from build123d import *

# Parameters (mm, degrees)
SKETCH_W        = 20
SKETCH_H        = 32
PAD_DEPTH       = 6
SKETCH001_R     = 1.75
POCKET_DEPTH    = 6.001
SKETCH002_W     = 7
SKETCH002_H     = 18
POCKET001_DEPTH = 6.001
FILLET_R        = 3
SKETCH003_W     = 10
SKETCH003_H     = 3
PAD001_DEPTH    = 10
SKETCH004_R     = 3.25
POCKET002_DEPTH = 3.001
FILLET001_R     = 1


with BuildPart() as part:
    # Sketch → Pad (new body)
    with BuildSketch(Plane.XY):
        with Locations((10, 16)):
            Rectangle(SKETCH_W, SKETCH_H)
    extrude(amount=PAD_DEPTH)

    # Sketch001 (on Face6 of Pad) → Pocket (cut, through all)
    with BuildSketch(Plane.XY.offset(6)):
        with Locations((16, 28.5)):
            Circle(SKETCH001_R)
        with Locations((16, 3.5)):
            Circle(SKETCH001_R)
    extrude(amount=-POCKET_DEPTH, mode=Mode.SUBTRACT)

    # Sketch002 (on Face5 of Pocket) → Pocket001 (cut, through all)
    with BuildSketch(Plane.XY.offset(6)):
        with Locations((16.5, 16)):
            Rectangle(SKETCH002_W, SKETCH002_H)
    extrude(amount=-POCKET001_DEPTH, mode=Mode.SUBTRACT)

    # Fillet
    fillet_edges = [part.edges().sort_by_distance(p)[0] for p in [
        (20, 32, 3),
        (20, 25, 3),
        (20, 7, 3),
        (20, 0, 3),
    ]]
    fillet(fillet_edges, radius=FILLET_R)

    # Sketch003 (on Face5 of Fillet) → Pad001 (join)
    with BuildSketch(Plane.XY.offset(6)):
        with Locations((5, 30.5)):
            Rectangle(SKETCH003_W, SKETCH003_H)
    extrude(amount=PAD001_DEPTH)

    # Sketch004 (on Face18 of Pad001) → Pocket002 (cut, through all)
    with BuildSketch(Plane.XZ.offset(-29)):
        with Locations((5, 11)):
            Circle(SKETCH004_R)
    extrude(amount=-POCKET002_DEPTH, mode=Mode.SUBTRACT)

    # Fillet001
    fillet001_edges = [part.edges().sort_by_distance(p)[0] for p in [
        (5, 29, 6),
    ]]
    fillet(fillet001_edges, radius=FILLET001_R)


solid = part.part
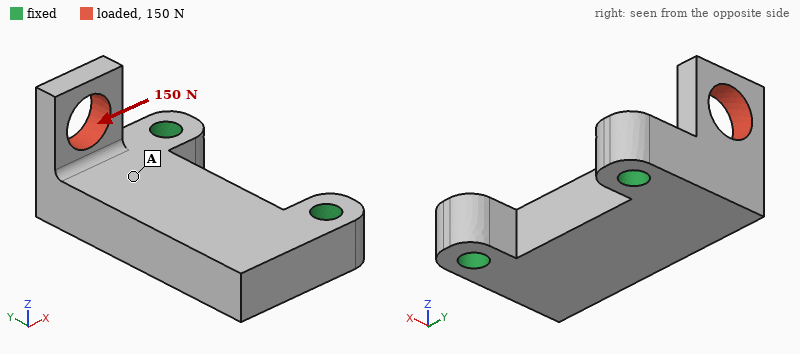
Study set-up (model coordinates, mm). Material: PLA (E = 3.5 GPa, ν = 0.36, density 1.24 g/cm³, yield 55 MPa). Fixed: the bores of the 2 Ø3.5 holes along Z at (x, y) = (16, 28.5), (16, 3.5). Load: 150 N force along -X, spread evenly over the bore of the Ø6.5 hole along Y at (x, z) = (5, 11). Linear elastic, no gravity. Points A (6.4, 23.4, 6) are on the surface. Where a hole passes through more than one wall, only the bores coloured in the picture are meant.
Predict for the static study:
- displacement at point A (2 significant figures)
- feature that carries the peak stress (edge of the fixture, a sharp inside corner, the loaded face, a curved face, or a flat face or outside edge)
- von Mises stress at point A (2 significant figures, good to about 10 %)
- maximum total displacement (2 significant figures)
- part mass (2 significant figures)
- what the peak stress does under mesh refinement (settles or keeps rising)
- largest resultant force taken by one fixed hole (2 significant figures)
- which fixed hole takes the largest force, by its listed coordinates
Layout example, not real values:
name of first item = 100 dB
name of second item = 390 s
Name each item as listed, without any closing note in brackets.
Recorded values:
displacement at point A = 0.075 mm
feature that carries the peak stress = a sharp inside corner
von Mises stress at point A = 6.3 MPa
maximum total displacement = 0.47 mm
part mass = 3.9 g
what the peak stress does under mesh refinement = keeps rising
largest resultant force taken by one fixed hole = 160 N
which fixed hole takes the largest force, by its listed coordinates = (16, 28.5)
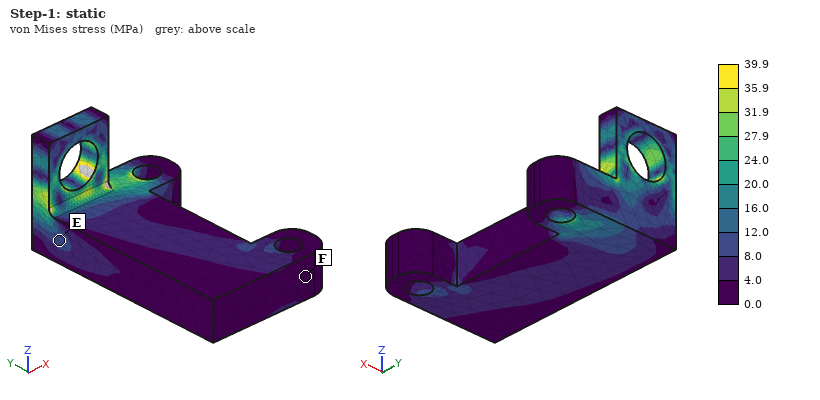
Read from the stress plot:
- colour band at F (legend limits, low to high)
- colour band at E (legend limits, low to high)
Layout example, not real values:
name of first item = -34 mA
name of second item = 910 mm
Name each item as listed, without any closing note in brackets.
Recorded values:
colour band at F = 0.0 to 4.0 MPa
colour band at E = 8.0 to 12.0 MPa
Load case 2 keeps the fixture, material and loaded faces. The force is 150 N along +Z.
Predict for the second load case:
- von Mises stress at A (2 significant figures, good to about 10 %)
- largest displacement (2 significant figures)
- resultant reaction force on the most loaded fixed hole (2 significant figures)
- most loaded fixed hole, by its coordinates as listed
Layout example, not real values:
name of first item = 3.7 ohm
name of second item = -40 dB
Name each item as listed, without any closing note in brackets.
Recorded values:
von Mises stress at A = 5.2 MPa
largest displacement = 0.28 mm
resultant reaction force on the most loaded fixed hole = 150 N
most loaded fixed hole, by its coordinates as listed = (16, 28.5)
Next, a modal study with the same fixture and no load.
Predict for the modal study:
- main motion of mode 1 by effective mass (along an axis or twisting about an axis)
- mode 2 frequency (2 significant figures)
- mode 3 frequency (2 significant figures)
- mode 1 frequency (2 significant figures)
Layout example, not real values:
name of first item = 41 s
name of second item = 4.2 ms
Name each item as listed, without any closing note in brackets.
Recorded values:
main motion of mode 1 by effective mass = along Z
mode 2 frequency = 5000 Hz
mode 3 frequency = 6800 Hz
mode 1 frequency = 3900 Hz
